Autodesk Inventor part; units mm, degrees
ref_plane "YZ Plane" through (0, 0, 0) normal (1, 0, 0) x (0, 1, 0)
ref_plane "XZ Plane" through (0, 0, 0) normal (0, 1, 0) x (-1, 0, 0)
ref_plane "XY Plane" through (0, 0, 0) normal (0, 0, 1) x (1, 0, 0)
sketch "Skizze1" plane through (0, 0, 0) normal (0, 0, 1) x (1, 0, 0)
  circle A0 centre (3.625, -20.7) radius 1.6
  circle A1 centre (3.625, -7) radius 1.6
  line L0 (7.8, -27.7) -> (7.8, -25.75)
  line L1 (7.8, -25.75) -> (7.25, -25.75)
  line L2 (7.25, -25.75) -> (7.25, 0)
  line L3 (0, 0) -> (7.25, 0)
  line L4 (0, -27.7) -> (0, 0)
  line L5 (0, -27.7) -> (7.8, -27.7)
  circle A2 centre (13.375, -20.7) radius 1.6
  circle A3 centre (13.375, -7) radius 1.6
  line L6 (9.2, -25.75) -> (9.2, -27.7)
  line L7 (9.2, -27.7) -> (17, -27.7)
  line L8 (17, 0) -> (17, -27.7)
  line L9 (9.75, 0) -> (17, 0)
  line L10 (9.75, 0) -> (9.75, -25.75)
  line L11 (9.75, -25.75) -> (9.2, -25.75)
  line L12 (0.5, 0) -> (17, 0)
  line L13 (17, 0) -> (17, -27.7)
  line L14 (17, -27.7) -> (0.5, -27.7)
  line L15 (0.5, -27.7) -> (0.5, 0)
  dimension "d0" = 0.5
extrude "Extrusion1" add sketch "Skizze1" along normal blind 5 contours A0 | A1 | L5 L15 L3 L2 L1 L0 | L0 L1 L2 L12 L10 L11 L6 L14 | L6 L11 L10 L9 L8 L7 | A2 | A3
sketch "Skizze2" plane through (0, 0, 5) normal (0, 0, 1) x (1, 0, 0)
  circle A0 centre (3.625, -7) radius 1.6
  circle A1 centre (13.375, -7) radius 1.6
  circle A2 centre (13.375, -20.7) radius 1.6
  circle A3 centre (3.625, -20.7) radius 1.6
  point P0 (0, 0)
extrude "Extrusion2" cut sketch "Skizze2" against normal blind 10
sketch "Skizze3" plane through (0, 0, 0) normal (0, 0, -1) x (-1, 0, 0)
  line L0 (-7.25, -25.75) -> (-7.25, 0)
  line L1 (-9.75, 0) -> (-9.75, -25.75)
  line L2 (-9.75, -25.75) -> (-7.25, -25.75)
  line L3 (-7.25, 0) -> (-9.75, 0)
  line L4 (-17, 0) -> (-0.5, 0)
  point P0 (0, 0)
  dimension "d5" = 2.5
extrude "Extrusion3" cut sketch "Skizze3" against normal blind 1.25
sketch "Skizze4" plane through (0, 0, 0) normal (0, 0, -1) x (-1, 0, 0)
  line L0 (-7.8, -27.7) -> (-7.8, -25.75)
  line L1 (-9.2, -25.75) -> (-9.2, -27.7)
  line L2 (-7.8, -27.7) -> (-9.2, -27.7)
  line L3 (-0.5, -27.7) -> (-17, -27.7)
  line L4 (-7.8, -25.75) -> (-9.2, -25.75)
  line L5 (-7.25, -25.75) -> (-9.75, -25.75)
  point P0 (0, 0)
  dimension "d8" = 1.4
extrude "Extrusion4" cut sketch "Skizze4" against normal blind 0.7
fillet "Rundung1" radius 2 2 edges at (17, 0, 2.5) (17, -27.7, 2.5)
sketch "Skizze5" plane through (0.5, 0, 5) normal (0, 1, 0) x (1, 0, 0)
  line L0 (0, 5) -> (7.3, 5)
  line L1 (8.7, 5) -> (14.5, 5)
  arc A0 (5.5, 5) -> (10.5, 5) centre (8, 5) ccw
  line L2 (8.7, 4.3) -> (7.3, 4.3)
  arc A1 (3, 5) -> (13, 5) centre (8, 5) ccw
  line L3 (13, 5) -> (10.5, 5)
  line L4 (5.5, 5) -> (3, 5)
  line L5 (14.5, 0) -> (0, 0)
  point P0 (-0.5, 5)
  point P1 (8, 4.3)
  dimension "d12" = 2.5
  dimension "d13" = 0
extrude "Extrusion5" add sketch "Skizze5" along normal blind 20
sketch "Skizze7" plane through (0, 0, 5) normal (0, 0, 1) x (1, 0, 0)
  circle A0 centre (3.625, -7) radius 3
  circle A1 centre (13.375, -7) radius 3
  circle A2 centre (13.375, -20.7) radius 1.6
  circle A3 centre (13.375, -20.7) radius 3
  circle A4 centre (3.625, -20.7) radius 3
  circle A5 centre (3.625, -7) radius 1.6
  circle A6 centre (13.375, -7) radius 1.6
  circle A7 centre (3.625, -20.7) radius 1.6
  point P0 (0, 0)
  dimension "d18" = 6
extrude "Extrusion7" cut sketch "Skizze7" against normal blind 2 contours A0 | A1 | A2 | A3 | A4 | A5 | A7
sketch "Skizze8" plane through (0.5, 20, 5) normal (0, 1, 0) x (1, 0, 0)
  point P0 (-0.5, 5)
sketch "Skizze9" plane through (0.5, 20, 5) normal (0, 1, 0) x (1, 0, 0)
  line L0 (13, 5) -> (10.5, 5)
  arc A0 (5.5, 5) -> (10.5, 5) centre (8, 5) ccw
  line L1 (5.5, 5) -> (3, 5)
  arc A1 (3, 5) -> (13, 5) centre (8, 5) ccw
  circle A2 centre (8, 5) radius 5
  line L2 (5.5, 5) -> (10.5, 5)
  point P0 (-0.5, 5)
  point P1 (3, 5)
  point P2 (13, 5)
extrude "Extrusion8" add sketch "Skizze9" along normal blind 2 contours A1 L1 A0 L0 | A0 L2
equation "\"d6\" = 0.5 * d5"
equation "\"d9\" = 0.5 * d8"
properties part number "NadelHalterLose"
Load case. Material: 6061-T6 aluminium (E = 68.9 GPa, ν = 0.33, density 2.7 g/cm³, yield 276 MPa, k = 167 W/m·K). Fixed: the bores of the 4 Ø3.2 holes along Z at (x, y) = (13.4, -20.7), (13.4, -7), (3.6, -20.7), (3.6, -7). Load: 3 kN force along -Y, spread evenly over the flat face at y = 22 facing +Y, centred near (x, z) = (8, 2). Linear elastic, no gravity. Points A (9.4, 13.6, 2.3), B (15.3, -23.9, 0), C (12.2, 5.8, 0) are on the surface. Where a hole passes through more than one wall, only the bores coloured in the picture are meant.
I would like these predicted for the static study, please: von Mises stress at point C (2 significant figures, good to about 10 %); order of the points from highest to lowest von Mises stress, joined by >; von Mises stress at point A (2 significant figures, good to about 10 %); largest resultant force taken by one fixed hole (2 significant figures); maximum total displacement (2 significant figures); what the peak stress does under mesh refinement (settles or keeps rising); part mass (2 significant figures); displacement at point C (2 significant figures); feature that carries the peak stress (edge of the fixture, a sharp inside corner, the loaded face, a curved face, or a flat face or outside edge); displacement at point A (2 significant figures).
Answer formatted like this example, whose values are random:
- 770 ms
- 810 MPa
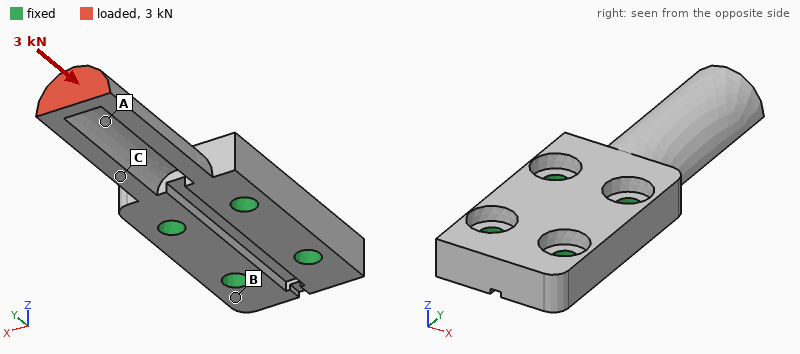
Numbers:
- 160 MPa
- C > A > B
- 110 MPa
- 1.4 kN
- 96 µm
- keeps rising
- 6.9 g
- 19 µm
- a sharp inside corner
- 34 µm
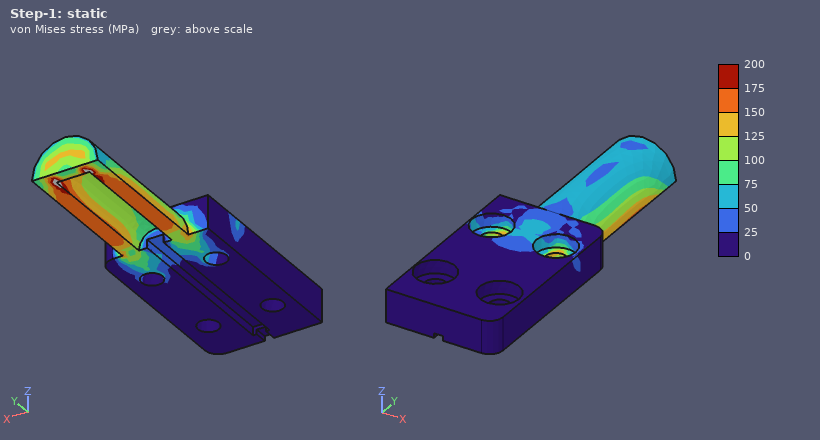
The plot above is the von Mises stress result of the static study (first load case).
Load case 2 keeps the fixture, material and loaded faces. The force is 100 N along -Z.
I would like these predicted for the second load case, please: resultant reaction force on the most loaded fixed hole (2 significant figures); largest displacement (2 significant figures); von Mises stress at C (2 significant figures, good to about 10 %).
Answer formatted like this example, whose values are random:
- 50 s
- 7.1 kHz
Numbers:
- 120 N
- 0.19 mm
- 82 MPa
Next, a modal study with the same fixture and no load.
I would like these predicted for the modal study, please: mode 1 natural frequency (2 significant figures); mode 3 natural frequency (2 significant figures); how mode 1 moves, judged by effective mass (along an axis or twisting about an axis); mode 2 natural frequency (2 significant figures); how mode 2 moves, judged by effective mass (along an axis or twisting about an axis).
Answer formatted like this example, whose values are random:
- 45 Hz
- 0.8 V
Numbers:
- 4800 Hz
- 17 kHz
- along Z
- 10000 Hz
- along X
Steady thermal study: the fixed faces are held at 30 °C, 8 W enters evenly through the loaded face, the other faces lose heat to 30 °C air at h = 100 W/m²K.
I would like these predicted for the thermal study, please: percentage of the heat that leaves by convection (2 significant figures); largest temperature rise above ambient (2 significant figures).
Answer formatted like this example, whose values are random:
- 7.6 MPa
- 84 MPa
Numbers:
- 17 %
- 37 K
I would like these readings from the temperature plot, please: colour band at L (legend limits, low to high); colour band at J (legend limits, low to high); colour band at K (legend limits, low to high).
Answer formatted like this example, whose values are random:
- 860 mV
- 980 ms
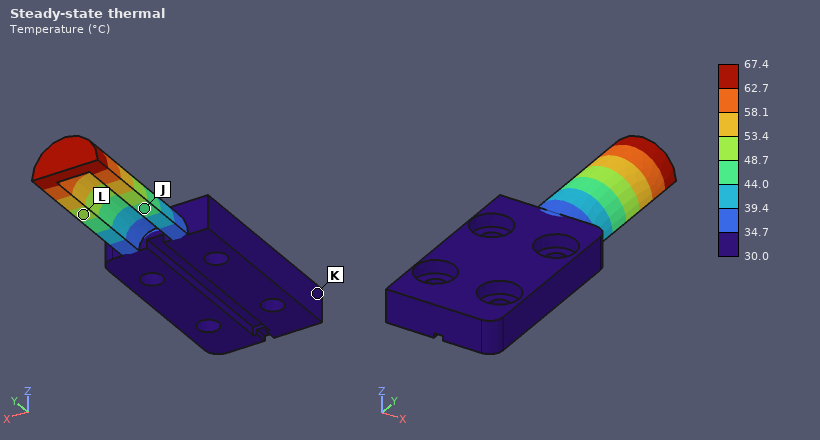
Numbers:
- 48.7 to 53.4 °C
- 44.0 to 48.7 °C
- 30.0 to 34.7 °C
